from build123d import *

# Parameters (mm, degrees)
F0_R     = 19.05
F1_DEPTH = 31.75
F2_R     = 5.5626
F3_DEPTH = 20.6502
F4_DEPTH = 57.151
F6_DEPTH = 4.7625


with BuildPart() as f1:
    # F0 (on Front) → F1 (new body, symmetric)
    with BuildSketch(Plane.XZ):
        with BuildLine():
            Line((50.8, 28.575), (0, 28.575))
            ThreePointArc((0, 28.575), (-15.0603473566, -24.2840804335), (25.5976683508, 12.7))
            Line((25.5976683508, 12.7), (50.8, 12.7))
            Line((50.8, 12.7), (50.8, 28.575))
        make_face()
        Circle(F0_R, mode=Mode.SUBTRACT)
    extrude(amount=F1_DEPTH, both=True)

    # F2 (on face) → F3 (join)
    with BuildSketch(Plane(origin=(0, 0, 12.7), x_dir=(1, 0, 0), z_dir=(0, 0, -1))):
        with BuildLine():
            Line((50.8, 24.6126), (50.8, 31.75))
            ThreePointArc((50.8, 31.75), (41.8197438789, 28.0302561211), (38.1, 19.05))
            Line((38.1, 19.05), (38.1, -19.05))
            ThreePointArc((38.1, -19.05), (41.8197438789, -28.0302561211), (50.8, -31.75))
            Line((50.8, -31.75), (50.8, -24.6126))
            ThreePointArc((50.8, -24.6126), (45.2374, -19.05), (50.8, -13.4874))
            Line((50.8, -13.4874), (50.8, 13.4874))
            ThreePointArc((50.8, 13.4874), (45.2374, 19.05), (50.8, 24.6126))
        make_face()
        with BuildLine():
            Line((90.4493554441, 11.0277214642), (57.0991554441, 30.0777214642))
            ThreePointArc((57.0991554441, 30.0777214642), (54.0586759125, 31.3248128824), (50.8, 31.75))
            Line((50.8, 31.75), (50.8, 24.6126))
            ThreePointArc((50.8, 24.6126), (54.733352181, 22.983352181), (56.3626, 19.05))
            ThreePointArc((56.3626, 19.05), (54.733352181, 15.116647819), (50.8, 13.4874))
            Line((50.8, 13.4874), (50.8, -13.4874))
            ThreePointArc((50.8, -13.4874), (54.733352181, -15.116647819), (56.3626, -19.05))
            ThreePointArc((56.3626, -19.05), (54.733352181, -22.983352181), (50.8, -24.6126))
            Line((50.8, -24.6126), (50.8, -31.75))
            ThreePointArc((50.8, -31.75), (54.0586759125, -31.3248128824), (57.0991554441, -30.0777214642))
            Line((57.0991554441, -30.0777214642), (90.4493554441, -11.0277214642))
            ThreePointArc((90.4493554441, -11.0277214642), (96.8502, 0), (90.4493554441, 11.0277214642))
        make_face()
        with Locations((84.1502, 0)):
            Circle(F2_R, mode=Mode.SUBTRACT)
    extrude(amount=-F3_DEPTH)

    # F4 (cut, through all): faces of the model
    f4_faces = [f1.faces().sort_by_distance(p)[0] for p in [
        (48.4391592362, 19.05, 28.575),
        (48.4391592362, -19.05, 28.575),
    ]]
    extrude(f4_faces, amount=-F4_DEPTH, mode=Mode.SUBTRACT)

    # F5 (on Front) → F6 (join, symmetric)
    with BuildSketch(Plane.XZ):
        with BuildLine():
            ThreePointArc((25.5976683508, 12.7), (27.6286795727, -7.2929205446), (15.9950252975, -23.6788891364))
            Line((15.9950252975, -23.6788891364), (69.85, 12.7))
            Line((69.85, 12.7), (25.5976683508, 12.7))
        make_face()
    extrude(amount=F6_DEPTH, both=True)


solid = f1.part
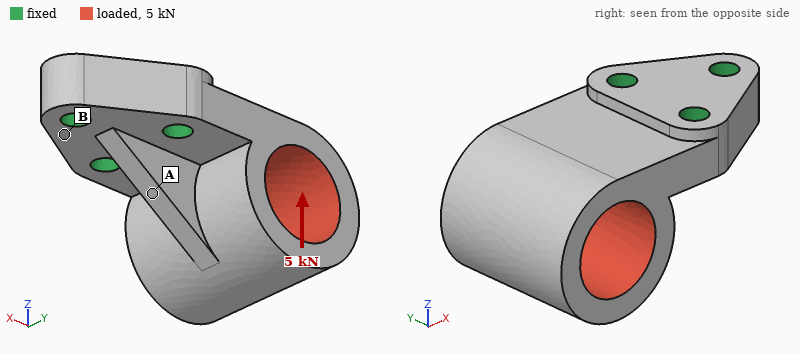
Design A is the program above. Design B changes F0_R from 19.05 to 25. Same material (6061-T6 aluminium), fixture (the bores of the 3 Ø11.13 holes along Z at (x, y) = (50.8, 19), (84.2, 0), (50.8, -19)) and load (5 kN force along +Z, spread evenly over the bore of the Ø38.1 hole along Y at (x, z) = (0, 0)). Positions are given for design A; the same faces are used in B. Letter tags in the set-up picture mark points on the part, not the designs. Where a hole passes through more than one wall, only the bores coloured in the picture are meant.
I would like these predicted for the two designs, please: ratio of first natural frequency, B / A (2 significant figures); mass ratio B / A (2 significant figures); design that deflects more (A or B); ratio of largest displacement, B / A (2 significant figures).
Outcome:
0.76
0.68
B
4.0
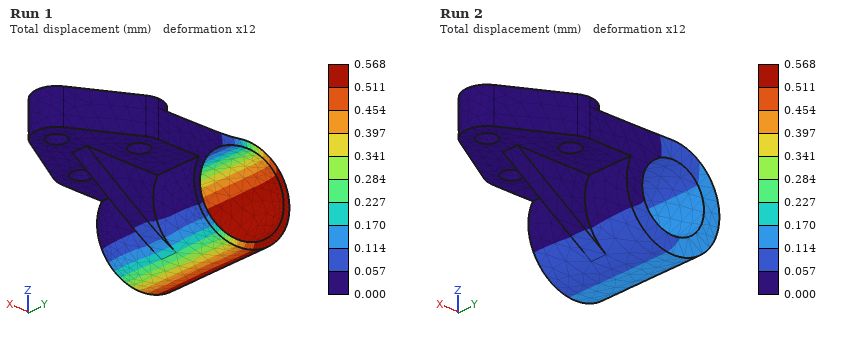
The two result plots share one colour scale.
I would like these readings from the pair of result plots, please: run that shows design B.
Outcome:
Run 1
